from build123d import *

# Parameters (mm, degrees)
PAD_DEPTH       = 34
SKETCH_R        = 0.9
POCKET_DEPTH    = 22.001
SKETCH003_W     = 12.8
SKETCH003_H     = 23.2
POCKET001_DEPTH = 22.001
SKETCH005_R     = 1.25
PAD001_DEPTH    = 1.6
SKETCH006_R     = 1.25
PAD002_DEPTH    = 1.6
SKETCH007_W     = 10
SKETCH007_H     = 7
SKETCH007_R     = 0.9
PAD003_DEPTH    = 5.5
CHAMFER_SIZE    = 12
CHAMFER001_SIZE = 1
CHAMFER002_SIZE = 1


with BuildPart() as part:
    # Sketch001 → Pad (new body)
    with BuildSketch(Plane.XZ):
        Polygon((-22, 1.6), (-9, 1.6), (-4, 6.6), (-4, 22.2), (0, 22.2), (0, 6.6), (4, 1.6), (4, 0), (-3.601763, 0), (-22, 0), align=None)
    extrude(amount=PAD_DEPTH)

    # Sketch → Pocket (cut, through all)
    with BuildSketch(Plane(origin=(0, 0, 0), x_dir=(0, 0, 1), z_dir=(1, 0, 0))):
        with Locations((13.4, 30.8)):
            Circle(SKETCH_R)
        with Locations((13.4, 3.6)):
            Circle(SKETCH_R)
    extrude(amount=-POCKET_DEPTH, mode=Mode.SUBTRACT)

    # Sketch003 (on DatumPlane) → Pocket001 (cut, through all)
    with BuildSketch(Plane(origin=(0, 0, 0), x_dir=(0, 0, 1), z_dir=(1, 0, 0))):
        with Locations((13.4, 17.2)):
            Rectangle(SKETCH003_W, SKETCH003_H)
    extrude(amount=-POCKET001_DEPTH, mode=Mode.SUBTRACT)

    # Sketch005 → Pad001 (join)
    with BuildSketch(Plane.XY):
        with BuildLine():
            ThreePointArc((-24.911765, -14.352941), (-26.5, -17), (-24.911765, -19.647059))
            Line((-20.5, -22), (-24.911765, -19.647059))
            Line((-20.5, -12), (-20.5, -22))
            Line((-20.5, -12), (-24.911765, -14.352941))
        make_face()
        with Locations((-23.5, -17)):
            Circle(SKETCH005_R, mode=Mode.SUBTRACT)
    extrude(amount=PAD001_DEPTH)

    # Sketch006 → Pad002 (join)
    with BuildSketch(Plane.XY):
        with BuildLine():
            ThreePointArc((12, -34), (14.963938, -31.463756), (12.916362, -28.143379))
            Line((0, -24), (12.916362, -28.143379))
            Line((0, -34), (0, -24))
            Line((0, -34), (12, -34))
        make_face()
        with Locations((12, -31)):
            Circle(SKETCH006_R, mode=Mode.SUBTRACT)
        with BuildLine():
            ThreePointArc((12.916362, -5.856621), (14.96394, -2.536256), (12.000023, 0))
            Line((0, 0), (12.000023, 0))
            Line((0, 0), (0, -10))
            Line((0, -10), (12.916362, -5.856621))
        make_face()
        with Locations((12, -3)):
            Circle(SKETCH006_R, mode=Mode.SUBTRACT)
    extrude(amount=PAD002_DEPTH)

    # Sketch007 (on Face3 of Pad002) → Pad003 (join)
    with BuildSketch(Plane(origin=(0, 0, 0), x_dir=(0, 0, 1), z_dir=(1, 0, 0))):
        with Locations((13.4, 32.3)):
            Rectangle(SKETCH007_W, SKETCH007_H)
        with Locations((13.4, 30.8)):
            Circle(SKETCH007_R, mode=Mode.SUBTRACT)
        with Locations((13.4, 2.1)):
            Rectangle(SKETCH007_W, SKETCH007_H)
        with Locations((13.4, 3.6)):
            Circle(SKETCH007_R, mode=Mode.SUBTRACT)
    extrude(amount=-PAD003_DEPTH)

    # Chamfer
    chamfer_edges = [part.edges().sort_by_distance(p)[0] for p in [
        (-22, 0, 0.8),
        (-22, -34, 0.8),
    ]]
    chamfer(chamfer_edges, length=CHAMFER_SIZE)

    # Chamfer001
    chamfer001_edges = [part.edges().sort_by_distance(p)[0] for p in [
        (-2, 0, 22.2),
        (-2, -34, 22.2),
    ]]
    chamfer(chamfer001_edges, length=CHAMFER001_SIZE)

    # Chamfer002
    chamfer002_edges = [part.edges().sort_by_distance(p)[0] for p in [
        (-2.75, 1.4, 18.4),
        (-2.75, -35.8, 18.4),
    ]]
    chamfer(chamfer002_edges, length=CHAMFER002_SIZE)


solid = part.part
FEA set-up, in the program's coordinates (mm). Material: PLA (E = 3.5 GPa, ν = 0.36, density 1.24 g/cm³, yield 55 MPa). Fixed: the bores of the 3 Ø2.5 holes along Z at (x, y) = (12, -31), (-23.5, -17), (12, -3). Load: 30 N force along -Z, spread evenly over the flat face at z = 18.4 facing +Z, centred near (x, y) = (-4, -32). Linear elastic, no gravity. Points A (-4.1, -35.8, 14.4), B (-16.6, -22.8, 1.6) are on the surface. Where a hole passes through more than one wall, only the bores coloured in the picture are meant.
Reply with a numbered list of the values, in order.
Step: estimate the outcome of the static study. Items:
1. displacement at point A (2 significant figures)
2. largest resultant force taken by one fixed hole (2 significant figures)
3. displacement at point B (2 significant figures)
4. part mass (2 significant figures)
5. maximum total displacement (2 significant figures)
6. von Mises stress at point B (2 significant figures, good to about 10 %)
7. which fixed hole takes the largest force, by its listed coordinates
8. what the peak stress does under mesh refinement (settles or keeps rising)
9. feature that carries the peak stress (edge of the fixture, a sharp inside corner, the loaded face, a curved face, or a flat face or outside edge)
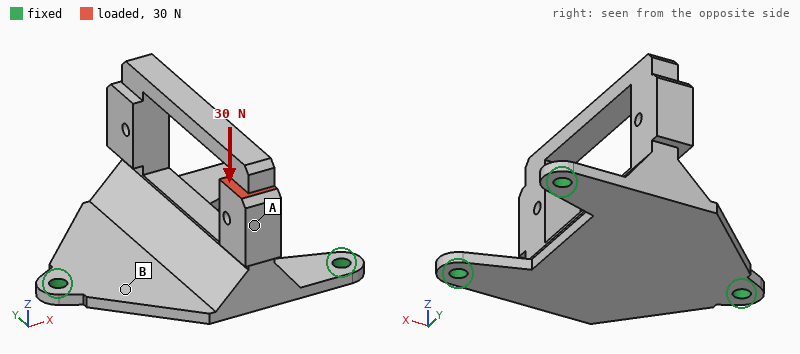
1. 0.35 mm
2. 28 N
3. 0.14 mm
4. 5.1 g
5. 0.40 mm
6. 4.9 MPa
7. (12, -31)
8. keeps rising
9. edge of the fixture
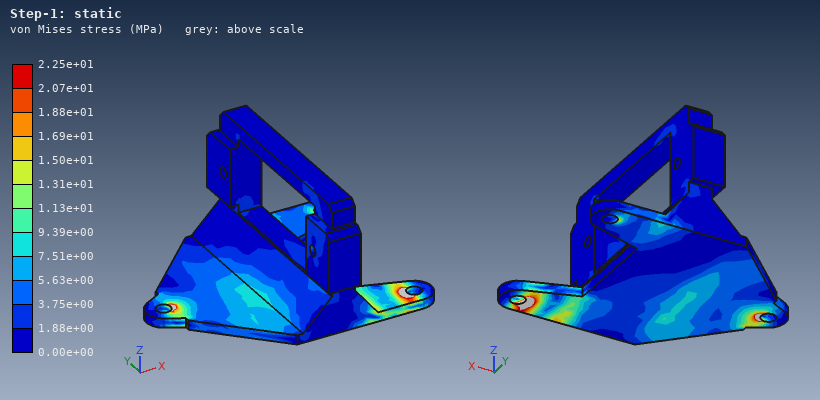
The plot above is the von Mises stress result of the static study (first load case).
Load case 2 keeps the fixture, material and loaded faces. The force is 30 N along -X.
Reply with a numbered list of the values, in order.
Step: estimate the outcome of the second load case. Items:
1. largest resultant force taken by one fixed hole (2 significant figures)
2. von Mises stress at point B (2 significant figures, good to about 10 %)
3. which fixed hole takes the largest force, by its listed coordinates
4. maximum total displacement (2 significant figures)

1. 27 N
2. 7.3 MPa
3. (-23.5, -17)
4. 0.64 mm
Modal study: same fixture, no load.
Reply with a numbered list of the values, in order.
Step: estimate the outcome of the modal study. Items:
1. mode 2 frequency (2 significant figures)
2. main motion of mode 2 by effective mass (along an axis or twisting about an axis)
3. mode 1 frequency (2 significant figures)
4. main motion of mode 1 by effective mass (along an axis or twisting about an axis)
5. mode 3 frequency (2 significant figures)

1. 1200 Hz
2. along Y
3. 1000 Hz
4. along Z
5. 1800 Hz
